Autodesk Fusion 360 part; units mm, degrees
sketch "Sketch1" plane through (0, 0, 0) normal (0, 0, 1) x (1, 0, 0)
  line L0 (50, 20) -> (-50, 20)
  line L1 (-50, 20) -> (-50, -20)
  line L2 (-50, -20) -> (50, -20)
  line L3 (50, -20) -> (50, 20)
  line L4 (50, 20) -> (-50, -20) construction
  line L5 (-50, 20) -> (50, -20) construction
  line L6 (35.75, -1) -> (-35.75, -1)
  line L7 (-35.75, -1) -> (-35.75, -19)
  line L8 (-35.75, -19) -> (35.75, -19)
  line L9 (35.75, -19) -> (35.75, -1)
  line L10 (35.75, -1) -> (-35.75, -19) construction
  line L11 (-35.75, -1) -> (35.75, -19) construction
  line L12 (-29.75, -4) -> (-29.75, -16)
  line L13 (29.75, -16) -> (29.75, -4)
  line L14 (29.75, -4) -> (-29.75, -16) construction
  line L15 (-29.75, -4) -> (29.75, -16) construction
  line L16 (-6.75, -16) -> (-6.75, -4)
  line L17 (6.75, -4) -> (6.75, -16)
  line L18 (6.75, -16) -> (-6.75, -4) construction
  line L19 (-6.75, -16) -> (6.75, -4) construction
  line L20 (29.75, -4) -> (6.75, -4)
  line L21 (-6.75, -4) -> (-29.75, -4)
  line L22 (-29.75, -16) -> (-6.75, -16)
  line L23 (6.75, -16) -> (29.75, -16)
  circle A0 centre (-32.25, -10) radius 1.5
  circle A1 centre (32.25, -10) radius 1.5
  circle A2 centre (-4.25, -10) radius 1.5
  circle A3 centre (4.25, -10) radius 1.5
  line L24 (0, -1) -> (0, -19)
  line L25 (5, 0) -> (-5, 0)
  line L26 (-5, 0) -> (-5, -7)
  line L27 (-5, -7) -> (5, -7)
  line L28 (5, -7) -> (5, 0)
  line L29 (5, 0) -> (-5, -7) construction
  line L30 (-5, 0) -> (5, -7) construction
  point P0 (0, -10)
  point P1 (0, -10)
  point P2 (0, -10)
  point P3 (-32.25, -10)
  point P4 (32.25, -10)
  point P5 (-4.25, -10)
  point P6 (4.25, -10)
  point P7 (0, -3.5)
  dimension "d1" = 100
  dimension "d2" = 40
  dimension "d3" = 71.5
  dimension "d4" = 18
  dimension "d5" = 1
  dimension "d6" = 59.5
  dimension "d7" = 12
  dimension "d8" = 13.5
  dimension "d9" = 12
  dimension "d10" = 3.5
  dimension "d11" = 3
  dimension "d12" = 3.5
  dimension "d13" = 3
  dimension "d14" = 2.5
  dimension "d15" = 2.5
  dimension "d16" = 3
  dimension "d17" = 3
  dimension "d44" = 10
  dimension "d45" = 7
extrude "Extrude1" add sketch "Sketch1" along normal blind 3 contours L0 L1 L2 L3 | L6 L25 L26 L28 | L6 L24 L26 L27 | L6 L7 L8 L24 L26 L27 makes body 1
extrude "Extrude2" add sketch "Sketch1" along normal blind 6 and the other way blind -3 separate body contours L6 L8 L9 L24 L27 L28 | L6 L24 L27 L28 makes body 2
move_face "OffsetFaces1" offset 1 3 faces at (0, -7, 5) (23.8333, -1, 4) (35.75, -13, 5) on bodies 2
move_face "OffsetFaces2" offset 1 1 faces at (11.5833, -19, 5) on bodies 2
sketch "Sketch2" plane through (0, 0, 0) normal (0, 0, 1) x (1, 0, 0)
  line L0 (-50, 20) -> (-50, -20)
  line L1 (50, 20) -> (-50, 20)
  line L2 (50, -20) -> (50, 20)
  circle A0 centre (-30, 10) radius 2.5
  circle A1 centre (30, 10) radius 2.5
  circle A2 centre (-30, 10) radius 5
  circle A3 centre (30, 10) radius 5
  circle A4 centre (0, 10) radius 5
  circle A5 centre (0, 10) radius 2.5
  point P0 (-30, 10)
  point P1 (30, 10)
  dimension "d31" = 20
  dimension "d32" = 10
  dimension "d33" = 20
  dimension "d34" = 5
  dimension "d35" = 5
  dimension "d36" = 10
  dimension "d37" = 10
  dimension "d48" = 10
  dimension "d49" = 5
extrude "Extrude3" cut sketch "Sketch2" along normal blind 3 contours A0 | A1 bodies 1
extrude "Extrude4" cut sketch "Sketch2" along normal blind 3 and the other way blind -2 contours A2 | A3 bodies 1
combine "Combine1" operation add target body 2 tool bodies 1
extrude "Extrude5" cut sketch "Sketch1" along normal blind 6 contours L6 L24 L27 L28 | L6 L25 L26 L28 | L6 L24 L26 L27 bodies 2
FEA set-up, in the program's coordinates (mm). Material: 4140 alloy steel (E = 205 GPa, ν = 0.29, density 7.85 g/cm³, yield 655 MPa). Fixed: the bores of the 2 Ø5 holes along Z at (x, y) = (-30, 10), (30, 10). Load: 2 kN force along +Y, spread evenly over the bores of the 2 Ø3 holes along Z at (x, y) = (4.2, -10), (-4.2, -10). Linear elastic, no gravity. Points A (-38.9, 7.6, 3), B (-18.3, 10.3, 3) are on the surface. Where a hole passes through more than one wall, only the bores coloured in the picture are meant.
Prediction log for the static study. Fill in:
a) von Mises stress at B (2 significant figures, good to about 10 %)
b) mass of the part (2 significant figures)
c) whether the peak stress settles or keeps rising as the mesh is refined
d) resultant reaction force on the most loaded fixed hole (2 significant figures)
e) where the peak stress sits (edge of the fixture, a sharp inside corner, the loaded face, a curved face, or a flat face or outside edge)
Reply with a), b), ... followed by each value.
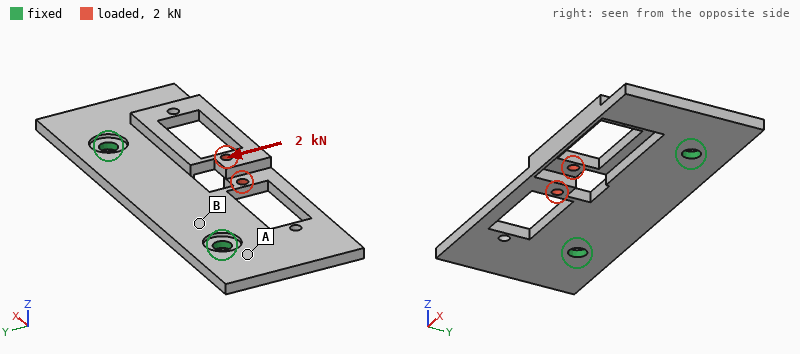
a) 58 MPa
b) 79 g
c) keeps rising
d) 1.0 kN
e) a sharp inside corner
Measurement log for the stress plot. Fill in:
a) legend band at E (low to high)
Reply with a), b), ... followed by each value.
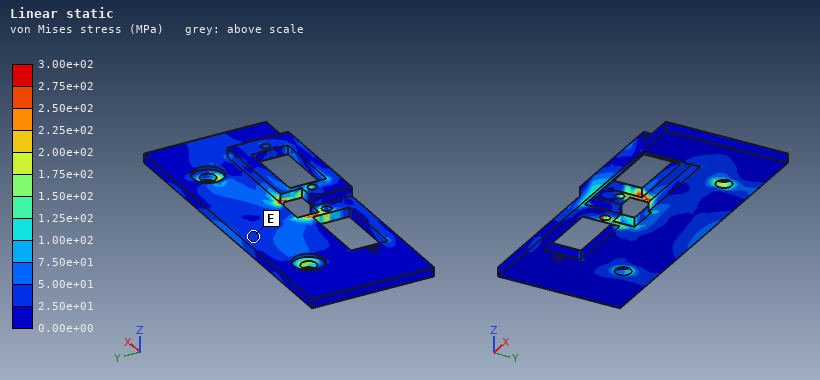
a) 2.50e+01 to 5.00e+01 MPa
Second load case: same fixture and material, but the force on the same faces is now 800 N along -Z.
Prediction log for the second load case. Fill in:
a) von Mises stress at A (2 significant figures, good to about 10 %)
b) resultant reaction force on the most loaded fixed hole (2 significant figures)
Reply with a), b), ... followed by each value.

a) 79 MPa
b) 600 N
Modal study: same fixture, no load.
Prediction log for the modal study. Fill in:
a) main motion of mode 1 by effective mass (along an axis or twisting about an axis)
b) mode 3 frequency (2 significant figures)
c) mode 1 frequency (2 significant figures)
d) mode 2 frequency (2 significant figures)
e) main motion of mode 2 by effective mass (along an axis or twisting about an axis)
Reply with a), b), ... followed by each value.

a) along Z
b) 2900 Hz
c) 1900 Hz
d) 2400 Hz
e) twisting about Y
